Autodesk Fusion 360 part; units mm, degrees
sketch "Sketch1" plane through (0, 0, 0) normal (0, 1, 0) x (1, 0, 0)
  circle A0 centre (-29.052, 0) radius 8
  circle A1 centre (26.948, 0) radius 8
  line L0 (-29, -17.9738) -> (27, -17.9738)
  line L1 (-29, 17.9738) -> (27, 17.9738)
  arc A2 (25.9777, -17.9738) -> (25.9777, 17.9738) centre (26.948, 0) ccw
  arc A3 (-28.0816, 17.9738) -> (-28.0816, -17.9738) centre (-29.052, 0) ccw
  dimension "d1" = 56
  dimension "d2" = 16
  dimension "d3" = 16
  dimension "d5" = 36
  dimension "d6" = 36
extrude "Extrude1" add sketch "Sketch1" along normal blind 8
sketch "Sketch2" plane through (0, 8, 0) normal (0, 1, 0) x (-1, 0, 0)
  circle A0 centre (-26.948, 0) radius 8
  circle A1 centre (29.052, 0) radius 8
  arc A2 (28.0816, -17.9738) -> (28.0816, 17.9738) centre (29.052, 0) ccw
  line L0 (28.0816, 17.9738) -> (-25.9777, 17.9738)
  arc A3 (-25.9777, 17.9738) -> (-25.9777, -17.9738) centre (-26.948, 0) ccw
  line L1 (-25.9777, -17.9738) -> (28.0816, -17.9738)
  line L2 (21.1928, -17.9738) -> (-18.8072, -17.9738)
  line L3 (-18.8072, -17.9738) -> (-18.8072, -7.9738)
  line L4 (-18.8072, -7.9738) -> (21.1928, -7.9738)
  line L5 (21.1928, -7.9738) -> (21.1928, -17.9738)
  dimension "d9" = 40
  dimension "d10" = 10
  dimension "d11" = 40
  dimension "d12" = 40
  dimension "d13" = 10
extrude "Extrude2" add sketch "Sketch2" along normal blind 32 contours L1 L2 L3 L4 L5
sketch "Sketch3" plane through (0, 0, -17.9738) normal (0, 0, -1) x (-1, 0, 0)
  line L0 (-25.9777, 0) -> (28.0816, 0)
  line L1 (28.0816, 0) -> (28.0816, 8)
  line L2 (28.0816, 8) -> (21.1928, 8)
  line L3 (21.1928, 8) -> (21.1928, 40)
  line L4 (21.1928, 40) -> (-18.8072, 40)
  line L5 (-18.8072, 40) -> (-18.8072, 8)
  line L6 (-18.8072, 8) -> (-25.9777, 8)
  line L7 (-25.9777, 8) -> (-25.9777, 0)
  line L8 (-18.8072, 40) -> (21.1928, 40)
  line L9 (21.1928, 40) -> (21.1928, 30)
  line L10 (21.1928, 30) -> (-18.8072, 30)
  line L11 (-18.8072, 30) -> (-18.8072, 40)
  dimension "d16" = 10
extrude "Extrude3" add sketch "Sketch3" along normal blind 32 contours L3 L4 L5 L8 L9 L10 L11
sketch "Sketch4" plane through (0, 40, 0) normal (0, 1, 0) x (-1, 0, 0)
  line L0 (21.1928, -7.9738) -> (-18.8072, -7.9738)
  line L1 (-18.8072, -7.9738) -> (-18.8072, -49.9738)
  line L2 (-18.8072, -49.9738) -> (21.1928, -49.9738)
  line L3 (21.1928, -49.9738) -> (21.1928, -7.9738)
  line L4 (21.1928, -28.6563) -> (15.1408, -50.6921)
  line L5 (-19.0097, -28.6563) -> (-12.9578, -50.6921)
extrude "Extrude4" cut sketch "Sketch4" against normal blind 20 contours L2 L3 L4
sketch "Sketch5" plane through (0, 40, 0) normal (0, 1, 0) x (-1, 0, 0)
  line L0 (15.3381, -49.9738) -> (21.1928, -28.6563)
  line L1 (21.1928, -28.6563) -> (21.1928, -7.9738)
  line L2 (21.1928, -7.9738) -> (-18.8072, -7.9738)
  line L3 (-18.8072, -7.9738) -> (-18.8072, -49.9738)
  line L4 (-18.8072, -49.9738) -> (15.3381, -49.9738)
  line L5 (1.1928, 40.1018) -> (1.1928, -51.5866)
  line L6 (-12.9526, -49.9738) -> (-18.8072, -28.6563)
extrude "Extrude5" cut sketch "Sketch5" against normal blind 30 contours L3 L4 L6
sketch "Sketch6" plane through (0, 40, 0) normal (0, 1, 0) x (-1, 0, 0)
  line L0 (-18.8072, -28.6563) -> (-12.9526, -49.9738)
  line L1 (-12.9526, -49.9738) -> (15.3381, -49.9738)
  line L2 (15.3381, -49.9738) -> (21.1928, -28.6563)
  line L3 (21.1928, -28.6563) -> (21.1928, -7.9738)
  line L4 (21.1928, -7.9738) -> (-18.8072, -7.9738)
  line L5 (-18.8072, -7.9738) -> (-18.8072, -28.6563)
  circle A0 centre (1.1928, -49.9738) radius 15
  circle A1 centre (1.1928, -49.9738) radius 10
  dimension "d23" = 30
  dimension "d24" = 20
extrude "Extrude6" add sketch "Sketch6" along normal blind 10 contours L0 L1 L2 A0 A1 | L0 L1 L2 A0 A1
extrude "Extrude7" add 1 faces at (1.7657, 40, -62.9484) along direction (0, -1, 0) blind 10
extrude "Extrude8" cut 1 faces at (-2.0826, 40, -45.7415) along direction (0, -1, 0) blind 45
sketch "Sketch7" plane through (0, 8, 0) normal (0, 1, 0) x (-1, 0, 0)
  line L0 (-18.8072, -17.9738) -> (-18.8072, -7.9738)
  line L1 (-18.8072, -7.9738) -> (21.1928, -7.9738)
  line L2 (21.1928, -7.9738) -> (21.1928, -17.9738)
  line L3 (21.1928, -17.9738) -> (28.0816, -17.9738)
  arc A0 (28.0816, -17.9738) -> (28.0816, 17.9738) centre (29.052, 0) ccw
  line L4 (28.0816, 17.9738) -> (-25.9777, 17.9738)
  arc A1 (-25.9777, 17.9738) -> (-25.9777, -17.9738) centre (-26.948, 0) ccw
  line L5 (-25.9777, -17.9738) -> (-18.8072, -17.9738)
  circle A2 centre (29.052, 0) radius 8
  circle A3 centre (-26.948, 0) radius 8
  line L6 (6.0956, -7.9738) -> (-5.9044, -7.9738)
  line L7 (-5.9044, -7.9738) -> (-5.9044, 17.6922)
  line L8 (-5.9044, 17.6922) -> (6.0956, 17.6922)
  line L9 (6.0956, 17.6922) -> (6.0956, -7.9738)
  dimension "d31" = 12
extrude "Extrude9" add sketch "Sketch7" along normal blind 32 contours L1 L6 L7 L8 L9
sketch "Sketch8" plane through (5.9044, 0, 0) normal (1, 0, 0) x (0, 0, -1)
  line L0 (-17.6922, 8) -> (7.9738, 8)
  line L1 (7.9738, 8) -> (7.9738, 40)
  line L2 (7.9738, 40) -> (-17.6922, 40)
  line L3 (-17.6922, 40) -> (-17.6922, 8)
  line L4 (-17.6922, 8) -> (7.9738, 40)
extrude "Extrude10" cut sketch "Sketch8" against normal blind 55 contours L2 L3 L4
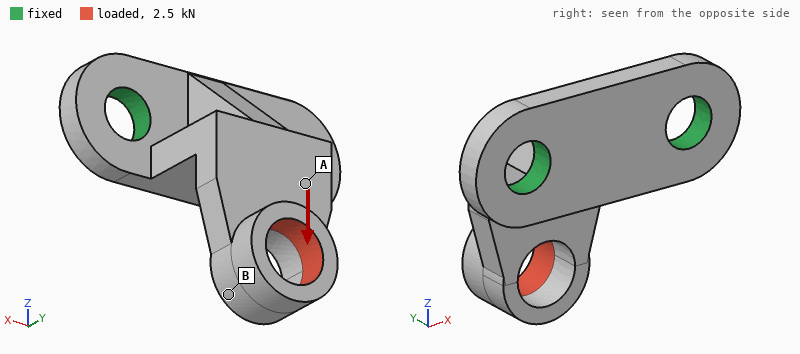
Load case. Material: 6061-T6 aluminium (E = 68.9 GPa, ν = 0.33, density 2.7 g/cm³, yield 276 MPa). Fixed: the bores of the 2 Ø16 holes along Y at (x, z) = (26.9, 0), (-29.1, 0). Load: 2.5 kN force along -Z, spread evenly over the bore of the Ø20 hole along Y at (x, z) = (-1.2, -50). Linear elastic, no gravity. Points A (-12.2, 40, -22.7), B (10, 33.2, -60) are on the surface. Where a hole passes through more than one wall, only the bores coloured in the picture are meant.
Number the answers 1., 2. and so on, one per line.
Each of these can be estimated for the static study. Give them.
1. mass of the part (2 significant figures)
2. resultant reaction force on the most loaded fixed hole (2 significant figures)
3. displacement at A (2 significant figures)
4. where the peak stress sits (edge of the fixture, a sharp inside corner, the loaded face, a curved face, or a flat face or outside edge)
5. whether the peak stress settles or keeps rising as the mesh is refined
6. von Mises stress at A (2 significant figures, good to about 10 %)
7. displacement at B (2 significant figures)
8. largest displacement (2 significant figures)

1. 150 g
2. 1.3 kN
3. 0.15 mm
4. edge of the fixture
5. keeps rising
6. 41 MPa
7. 0.35 mm
8. 0.45 mm
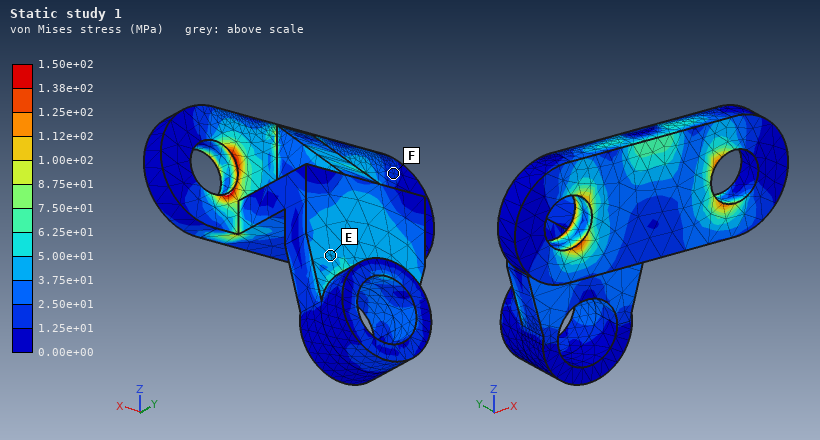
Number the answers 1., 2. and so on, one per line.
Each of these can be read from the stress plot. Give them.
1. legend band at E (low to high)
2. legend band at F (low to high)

1. 3.75e+01 to 5.00e+01 MPa
2. 1.25e+01 to 2.50e+01 MPa
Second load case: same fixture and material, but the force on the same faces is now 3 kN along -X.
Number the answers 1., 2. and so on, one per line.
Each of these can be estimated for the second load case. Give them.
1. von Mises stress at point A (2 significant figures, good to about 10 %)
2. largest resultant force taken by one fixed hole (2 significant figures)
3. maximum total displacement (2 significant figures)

1. 17 MPa
2. 4.2 kN
3. 0.33 mm
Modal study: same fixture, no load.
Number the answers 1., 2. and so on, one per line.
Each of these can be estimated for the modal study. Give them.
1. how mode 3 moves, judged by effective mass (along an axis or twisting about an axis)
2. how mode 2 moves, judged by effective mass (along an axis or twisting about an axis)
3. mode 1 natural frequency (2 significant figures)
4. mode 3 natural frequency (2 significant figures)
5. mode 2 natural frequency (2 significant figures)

1. along Z
2. along X
3. 2000 Hz
4. 5100 Hz
5. 3300 Hz
